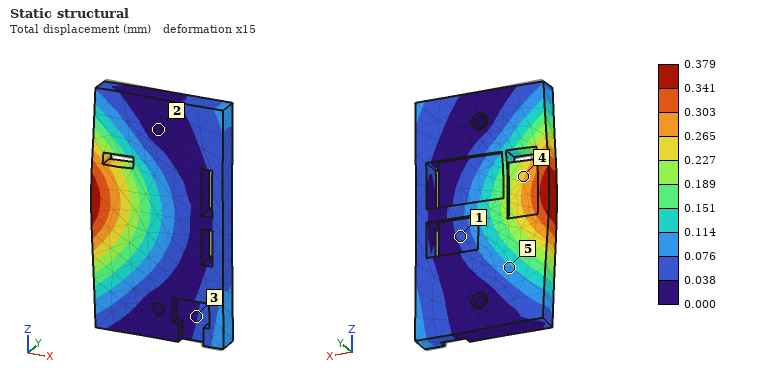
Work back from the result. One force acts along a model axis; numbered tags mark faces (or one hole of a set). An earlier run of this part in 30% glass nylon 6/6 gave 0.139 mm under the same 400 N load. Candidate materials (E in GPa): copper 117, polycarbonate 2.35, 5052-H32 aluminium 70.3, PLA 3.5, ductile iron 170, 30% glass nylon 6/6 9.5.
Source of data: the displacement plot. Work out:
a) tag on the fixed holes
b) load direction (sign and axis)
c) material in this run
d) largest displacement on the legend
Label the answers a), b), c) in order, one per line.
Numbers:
a) 2
b) -Y
c) PLA
d) 0.379 mm
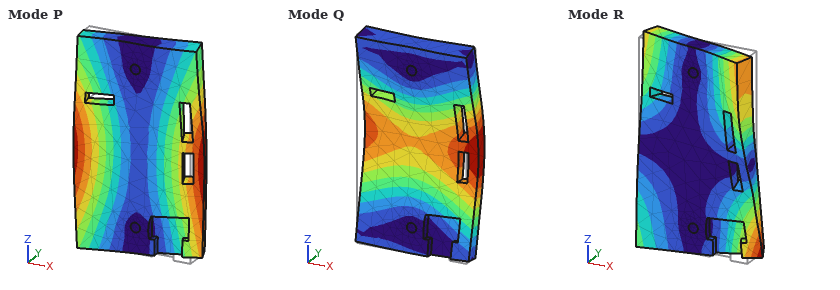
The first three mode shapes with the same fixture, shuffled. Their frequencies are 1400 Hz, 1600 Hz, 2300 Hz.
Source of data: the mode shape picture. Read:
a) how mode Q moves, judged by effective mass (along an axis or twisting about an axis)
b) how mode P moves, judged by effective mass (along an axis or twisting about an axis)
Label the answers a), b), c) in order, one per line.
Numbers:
a) along Y
b) twisting about Z
